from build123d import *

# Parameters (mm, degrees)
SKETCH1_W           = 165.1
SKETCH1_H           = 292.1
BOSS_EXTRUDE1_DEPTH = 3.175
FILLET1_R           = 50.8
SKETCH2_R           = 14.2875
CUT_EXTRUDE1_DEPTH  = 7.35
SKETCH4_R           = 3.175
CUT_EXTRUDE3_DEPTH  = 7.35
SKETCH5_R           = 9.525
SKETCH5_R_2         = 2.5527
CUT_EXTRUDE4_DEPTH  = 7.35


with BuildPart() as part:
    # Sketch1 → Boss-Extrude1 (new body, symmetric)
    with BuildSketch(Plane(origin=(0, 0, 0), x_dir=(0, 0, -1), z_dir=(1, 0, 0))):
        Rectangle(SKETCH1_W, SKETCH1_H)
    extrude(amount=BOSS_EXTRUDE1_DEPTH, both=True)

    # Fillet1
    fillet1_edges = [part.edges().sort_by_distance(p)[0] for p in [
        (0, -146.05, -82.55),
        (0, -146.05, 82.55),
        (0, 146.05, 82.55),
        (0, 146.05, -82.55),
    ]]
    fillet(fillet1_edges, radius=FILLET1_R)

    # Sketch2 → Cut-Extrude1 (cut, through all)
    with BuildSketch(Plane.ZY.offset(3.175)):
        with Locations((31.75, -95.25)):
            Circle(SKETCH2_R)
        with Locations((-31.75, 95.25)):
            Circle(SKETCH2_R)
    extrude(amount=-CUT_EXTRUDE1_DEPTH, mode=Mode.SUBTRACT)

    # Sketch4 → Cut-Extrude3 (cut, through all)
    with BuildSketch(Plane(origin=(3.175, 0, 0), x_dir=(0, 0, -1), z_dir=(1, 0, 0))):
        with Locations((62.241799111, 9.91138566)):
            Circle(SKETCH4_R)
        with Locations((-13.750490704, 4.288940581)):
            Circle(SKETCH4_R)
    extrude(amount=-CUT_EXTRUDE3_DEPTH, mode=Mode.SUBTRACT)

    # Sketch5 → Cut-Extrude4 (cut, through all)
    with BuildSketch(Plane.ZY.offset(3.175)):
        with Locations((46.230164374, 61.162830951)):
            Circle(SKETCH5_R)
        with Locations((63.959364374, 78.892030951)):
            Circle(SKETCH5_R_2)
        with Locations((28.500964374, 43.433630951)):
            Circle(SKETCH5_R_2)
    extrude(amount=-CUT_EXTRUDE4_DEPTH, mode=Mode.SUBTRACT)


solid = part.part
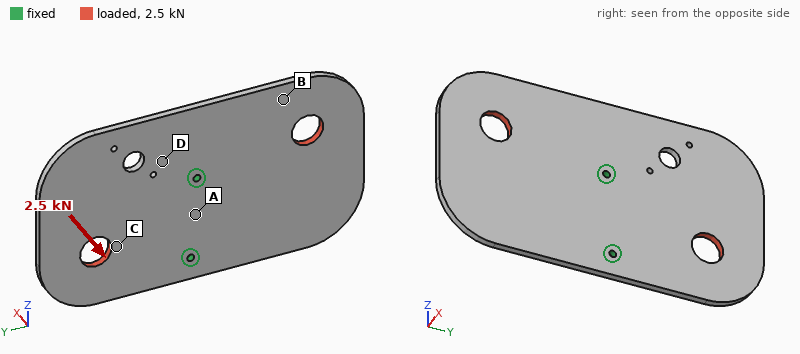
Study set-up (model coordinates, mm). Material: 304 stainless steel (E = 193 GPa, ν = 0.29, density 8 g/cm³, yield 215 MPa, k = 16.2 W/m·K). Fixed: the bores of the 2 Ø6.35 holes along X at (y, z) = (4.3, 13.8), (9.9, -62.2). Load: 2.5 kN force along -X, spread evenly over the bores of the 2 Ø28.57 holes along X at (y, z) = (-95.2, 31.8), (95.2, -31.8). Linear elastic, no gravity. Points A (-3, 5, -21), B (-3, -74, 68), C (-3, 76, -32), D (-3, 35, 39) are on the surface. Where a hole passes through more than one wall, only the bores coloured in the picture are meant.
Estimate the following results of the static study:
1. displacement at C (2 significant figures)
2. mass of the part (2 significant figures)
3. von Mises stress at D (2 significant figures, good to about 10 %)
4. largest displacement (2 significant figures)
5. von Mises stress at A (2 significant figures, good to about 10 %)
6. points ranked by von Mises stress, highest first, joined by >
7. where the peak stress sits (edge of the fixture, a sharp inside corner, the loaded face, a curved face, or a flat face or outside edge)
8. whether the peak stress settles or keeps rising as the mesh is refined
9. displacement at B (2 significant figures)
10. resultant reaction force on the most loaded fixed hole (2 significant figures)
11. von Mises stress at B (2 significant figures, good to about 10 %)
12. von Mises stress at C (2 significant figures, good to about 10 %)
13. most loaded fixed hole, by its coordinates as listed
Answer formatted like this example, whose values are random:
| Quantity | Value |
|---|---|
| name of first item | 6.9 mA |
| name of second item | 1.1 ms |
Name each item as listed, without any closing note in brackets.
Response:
| Quantity | Value |
|---|---|
| displacement at C | 0.30 mm |
| mass of the part | 2.3 kg |
| von Mises stress at D | 60 MPa |
| largest displacement | 1.3 mm |
| von Mises stress at A | 91 MPa |
| points ranked by von Mises stress, highest first, joined by > | A > D > C > B |
| where the peak stress sits | edge of the fixture |
| whether the peak stress settles or keeps rising as the mesh is refined | keeps rising |
| displacement at B | 0.60 mm |
| resultant reaction force on the most loaded fixed hole | 1.9 kN |
| von Mises stress at B | 22 MPa |
| von Mises stress at C | 38 MPa |
| most loaded fixed hole, by its coordinates as listed | (4.3, 13.8) |
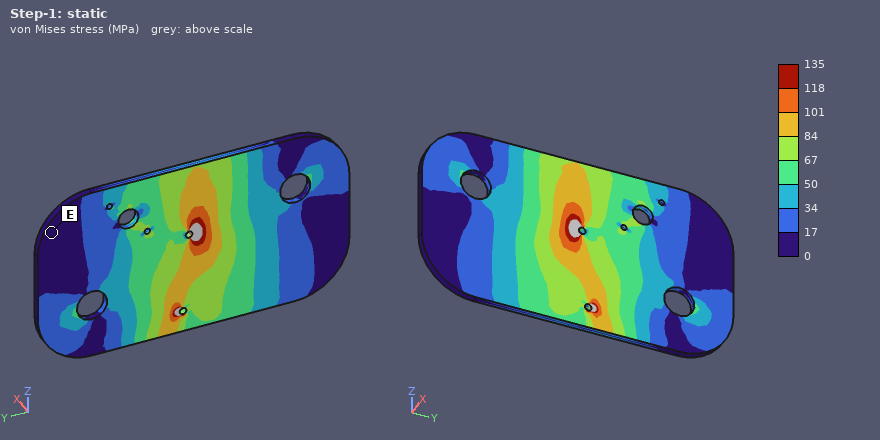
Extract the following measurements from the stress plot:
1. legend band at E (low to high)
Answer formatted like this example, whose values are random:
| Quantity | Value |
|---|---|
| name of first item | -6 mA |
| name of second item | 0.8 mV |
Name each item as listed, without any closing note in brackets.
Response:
| Quantity | Value |
|---|---|
| legend band at E | 0 to 17 MPa |
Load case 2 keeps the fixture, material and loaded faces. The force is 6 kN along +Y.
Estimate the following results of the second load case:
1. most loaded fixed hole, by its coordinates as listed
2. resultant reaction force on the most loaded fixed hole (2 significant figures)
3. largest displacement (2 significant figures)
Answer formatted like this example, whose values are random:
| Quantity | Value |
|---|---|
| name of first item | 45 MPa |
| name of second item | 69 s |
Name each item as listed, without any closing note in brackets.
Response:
| Quantity | Value |
|---|---|
| most loaded fixed hole, by its coordinates as listed | (4.3, 13.8) |
| resultant reaction force on the most loaded fixed hole | 4.9 kN |
| largest displacement | 9.5 µm |
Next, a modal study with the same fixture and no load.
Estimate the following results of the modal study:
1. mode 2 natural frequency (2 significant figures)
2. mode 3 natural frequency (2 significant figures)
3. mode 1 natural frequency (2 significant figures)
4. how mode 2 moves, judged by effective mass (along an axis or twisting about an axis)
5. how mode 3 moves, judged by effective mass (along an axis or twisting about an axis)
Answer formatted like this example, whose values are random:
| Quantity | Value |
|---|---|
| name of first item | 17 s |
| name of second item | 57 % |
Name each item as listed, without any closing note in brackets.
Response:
| Quantity | Value |
|---|---|
| mode 2 natural frequency | 270 Hz |
| mode 3 natural frequency | 490 Hz |
| mode 1 natural frequency | 200 Hz |
| how mode 2 moves, judged by effective mass | along X |
| how mode 3 moves, judged by effective mass | twisting about Y |
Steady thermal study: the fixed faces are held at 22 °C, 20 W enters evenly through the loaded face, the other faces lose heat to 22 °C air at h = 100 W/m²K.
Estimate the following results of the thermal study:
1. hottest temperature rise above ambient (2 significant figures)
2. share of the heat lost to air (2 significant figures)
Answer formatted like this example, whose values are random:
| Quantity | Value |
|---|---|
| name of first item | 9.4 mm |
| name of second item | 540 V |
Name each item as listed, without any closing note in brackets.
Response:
| Quantity | Value |
|---|---|
| hottest temperature rise above ambient | 16 K |
| share of the heat lost to air | 99 % |
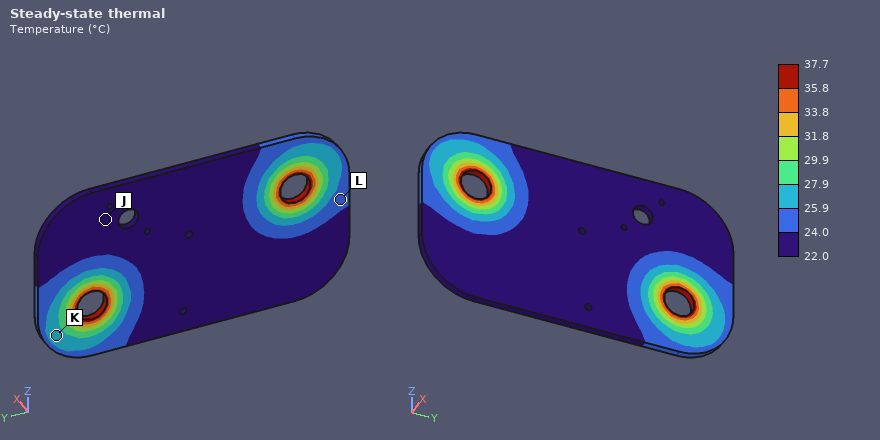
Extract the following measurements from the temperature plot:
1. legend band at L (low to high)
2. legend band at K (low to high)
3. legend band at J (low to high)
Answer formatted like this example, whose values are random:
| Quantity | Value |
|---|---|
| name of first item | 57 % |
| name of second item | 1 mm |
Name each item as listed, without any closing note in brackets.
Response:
| Quantity | Value |
|---|---|
| legend band at L | 24.0 to 25.9 °C |
| legend band at K | 25.9 to 27.9 °C |
| legend band at J | 22.0 to 24.0 °C |
